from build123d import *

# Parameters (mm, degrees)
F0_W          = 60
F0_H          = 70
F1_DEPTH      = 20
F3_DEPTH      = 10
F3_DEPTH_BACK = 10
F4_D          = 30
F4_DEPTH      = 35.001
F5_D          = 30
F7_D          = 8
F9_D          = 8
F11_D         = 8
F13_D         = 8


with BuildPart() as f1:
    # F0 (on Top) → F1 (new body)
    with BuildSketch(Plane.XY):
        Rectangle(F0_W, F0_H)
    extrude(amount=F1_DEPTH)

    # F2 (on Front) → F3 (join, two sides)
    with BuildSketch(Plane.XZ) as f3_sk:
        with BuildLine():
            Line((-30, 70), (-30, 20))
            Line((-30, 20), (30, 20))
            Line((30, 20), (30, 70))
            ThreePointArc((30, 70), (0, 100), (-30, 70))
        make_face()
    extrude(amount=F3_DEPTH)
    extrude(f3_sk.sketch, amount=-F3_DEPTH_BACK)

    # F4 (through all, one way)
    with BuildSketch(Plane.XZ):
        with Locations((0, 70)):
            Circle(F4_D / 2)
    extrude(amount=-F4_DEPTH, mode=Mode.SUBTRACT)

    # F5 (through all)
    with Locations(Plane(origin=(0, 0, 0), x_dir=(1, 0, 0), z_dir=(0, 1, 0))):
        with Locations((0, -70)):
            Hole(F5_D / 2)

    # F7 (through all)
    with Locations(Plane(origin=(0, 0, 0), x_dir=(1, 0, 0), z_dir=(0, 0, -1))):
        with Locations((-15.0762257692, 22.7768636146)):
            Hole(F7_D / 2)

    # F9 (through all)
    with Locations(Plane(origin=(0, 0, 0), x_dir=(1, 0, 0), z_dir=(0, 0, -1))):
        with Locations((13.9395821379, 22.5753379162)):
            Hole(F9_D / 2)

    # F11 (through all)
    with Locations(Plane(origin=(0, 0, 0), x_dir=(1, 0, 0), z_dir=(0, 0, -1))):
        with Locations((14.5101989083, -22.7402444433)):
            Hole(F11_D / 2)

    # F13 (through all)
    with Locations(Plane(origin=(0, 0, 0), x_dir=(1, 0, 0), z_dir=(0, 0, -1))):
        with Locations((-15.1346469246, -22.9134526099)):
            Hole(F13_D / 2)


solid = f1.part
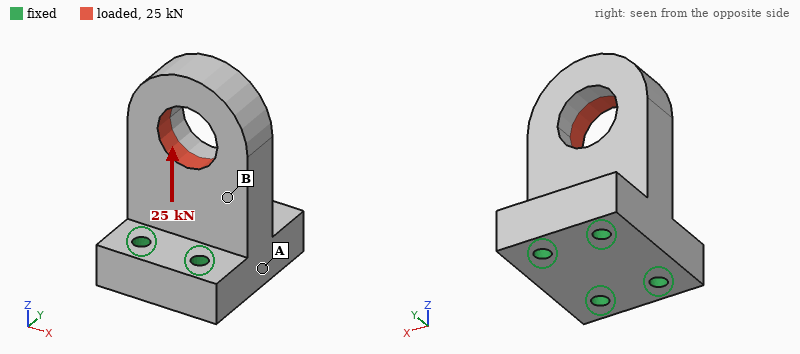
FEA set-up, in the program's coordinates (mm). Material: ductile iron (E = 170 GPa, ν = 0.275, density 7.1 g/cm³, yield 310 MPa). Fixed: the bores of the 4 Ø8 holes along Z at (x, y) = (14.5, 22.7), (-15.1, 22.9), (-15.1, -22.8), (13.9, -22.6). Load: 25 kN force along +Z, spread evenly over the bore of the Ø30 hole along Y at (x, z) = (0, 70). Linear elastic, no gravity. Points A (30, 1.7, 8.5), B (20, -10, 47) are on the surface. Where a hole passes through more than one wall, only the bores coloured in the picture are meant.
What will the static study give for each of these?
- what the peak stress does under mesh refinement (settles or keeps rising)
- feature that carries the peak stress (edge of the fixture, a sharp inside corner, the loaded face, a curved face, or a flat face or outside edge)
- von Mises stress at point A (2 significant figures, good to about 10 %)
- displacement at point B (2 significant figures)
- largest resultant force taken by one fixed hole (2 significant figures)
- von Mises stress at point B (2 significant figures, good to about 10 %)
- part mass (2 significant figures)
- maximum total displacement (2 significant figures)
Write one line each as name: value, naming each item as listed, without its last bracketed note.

what the peak stress does under mesh refinement: keeps rising
feature that carries the peak stress: edge of the fixture
von Mises stress at point A: 14 MPa
displacement at point B: 18 µm
largest resultant force taken by one fixed hole: 8.2 kN
von Mises stress at point B: 60 MPa
part mass: 1.1 kg
maximum total displacement: 78 µm
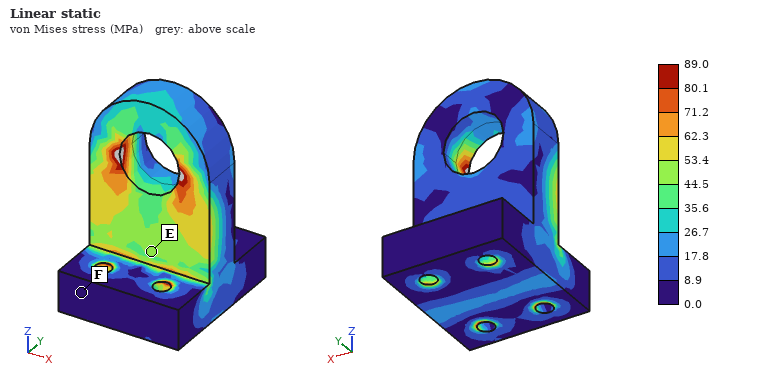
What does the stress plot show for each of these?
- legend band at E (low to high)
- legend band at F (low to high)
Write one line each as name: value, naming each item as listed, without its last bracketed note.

legend band at E: 44.5 to 53.4 MPa
legend band at F: 0.0 to 8.9 MPa
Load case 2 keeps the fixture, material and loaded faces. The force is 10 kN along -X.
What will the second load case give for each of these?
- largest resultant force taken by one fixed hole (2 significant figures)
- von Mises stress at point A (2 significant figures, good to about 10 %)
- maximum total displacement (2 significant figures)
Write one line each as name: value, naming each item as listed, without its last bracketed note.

largest resultant force taken by one fixed hole: 7.8 kN
von Mises stress at point A: 21 MPa
maximum total displacement: 62 µm
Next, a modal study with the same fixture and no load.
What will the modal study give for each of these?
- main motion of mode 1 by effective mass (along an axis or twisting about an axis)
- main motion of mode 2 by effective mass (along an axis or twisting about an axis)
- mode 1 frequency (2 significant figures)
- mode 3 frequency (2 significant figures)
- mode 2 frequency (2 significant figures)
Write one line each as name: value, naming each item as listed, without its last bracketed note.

main motion of mode 1 by effective mass: along Y
main motion of mode 2 by effective mass: along X
mode 1 frequency: 2500 Hz
mode 3 frequency: 6200 Hz
mode 2 frequency: 4100 Hz
